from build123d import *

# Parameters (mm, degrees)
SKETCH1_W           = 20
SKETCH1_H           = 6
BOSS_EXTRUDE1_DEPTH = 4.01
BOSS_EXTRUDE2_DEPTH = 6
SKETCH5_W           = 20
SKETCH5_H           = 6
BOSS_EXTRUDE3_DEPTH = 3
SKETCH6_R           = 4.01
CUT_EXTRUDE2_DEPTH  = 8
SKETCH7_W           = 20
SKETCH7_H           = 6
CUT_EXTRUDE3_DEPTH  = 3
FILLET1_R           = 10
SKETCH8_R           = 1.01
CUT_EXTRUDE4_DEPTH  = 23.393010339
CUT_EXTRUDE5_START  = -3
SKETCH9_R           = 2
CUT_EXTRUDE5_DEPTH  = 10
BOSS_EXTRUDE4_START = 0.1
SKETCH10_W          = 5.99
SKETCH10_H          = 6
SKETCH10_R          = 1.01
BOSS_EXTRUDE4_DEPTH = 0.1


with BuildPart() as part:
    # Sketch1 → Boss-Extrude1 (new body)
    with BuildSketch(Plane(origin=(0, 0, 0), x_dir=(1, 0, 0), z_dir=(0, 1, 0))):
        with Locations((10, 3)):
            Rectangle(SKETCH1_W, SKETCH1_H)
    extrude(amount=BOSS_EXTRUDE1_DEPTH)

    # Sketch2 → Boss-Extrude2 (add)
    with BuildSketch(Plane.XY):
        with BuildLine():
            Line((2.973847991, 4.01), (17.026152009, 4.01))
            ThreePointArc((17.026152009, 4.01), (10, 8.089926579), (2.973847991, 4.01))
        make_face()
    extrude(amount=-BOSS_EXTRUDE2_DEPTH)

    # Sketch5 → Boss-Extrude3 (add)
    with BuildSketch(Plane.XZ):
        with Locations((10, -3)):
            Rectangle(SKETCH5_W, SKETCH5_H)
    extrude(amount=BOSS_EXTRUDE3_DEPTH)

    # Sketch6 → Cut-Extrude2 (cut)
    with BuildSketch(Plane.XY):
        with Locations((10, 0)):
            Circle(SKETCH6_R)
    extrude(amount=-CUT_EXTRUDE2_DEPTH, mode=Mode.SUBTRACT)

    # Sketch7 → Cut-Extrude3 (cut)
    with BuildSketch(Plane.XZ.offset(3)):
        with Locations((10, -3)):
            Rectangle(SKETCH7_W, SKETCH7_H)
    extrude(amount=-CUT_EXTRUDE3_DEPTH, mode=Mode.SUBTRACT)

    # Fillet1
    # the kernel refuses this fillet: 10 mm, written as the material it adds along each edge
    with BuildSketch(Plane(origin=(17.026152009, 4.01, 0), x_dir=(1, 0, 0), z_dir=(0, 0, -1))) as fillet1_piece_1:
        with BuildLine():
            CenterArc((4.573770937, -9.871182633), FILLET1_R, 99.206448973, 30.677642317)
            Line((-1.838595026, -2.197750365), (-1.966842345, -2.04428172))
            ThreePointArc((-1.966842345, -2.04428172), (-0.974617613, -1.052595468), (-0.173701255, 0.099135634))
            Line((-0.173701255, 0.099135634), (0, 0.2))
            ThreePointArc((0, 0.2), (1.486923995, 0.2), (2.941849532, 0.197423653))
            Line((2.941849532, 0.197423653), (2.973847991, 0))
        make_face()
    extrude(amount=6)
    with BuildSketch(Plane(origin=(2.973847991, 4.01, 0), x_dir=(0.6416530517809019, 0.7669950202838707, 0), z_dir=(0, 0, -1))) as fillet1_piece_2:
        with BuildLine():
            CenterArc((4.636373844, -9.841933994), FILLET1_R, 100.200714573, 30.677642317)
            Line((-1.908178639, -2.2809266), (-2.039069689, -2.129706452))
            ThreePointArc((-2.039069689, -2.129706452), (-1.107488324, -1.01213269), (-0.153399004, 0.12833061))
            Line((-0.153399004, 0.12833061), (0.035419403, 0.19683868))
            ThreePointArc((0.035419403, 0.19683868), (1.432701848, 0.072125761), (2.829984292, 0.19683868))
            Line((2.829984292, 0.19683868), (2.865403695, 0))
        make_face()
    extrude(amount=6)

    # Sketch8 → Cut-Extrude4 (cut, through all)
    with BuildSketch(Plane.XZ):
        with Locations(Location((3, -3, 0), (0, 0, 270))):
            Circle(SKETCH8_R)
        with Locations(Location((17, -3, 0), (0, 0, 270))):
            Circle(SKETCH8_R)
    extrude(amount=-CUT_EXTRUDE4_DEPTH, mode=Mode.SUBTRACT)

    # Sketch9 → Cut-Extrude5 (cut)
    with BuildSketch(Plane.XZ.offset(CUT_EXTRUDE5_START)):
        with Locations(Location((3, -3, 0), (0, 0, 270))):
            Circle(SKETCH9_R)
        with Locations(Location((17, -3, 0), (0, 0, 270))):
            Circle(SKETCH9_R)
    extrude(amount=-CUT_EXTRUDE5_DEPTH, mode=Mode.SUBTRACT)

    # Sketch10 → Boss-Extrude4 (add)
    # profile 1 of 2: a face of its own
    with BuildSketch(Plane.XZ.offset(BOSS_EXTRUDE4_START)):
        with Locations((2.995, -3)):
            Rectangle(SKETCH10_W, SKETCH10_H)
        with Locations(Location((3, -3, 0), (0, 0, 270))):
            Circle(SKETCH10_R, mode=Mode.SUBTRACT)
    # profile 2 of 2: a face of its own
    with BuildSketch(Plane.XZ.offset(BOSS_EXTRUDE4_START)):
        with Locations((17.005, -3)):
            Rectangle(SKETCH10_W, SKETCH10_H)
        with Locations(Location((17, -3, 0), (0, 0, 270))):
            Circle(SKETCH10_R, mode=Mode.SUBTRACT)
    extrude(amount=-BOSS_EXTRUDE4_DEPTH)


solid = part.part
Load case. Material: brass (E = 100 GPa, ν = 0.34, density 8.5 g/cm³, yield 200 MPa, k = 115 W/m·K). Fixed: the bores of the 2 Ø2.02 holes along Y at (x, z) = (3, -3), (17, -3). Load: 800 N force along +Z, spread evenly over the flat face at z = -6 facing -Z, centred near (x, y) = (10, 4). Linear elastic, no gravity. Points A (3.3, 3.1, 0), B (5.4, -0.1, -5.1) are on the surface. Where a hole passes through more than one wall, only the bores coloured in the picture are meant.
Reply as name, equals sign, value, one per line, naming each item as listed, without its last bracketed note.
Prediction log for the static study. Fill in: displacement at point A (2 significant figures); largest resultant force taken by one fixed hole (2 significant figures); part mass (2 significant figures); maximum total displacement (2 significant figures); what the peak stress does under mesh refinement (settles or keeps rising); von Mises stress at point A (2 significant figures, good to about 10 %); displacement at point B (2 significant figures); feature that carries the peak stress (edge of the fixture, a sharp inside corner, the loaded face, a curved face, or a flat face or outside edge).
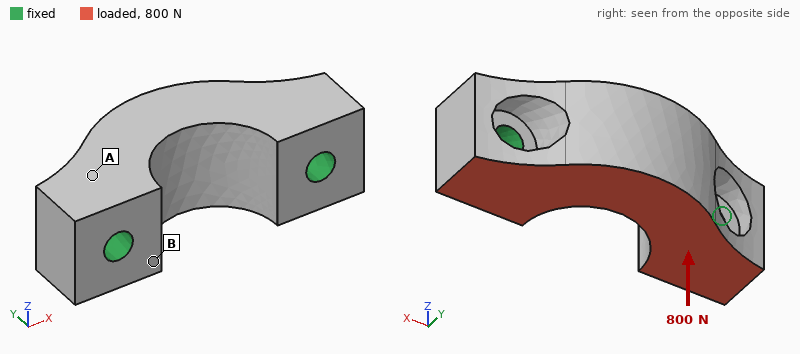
displacement at point A = 2.2 µm
largest resultant force taken by one fixed hole = 400 N
part mass = 4.5 g
maximum total displacement = 9.5 µm
what the peak stress does under mesh refinement = keeps rising
von Mises stress at point A = 45 MPa
displacement at point B = 1.6 µm
feature that carries the peak stress = edge of the fixture
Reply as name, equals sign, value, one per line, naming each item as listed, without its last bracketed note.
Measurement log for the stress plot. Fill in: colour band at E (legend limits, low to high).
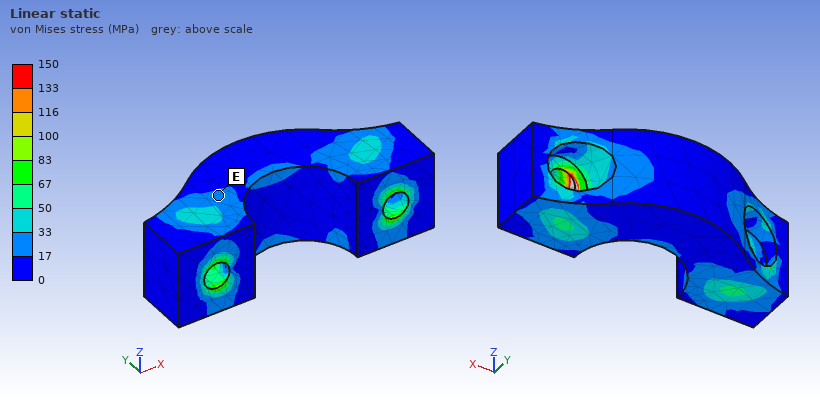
colour band at E = 17 to 33 MPa
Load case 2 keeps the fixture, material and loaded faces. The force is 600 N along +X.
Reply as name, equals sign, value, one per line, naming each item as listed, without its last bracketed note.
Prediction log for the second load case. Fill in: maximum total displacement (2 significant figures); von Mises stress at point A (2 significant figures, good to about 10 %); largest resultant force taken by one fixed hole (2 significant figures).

maximum total displacement = 2.6 µm
von Mises stress at point A = 12 MPa
largest resultant force taken by one fixed hole = 320 N
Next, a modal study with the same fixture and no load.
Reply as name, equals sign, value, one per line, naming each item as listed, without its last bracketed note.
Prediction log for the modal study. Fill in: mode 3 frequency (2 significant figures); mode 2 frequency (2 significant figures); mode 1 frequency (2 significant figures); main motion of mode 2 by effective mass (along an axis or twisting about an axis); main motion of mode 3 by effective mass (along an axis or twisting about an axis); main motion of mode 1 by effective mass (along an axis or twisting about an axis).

mode 3 frequency = 59 kHz
mode 2 frequency = 56 kHz
mode 1 frequency = 26 kHz
main motion of mode 2 by effective mass = along Y
main motion of mode 3 by effective mass = along X
main motion of mode 1 by effective mass = along Z
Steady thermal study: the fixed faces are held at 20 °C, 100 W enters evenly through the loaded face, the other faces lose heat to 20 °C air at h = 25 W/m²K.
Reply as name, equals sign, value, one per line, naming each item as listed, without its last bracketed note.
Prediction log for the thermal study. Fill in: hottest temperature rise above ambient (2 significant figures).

hottest temperature rise above ambient = 86 K
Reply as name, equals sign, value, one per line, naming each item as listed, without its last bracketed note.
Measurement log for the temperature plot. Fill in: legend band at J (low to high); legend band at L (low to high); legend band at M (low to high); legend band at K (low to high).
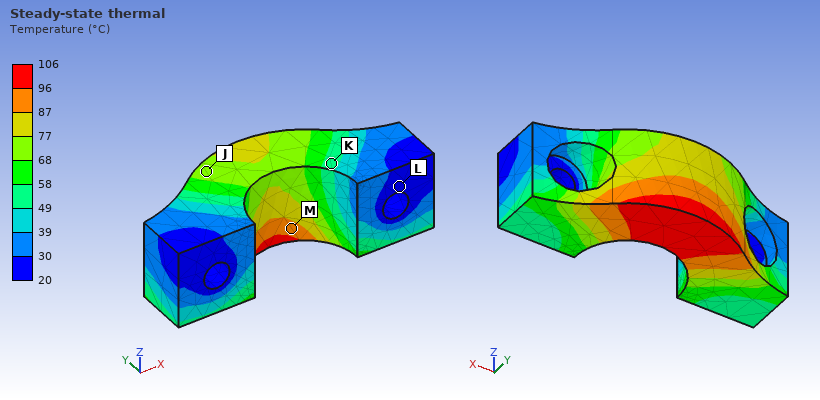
legend band at J = 68 to 77 °C
legend band at L = 20 to 30 °C
legend band at M = 87 to 96 °C
legend band at K = 49 to 58 °C
